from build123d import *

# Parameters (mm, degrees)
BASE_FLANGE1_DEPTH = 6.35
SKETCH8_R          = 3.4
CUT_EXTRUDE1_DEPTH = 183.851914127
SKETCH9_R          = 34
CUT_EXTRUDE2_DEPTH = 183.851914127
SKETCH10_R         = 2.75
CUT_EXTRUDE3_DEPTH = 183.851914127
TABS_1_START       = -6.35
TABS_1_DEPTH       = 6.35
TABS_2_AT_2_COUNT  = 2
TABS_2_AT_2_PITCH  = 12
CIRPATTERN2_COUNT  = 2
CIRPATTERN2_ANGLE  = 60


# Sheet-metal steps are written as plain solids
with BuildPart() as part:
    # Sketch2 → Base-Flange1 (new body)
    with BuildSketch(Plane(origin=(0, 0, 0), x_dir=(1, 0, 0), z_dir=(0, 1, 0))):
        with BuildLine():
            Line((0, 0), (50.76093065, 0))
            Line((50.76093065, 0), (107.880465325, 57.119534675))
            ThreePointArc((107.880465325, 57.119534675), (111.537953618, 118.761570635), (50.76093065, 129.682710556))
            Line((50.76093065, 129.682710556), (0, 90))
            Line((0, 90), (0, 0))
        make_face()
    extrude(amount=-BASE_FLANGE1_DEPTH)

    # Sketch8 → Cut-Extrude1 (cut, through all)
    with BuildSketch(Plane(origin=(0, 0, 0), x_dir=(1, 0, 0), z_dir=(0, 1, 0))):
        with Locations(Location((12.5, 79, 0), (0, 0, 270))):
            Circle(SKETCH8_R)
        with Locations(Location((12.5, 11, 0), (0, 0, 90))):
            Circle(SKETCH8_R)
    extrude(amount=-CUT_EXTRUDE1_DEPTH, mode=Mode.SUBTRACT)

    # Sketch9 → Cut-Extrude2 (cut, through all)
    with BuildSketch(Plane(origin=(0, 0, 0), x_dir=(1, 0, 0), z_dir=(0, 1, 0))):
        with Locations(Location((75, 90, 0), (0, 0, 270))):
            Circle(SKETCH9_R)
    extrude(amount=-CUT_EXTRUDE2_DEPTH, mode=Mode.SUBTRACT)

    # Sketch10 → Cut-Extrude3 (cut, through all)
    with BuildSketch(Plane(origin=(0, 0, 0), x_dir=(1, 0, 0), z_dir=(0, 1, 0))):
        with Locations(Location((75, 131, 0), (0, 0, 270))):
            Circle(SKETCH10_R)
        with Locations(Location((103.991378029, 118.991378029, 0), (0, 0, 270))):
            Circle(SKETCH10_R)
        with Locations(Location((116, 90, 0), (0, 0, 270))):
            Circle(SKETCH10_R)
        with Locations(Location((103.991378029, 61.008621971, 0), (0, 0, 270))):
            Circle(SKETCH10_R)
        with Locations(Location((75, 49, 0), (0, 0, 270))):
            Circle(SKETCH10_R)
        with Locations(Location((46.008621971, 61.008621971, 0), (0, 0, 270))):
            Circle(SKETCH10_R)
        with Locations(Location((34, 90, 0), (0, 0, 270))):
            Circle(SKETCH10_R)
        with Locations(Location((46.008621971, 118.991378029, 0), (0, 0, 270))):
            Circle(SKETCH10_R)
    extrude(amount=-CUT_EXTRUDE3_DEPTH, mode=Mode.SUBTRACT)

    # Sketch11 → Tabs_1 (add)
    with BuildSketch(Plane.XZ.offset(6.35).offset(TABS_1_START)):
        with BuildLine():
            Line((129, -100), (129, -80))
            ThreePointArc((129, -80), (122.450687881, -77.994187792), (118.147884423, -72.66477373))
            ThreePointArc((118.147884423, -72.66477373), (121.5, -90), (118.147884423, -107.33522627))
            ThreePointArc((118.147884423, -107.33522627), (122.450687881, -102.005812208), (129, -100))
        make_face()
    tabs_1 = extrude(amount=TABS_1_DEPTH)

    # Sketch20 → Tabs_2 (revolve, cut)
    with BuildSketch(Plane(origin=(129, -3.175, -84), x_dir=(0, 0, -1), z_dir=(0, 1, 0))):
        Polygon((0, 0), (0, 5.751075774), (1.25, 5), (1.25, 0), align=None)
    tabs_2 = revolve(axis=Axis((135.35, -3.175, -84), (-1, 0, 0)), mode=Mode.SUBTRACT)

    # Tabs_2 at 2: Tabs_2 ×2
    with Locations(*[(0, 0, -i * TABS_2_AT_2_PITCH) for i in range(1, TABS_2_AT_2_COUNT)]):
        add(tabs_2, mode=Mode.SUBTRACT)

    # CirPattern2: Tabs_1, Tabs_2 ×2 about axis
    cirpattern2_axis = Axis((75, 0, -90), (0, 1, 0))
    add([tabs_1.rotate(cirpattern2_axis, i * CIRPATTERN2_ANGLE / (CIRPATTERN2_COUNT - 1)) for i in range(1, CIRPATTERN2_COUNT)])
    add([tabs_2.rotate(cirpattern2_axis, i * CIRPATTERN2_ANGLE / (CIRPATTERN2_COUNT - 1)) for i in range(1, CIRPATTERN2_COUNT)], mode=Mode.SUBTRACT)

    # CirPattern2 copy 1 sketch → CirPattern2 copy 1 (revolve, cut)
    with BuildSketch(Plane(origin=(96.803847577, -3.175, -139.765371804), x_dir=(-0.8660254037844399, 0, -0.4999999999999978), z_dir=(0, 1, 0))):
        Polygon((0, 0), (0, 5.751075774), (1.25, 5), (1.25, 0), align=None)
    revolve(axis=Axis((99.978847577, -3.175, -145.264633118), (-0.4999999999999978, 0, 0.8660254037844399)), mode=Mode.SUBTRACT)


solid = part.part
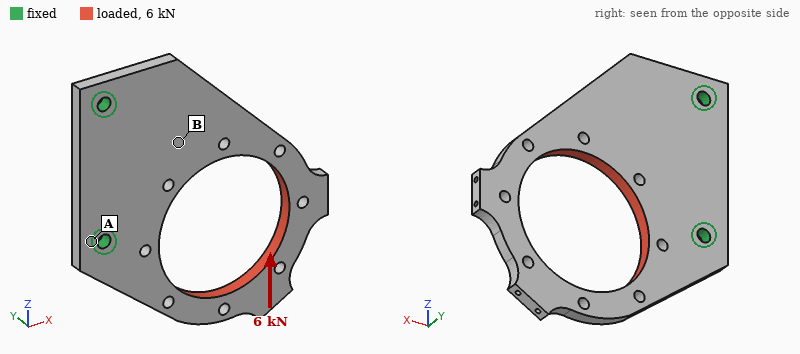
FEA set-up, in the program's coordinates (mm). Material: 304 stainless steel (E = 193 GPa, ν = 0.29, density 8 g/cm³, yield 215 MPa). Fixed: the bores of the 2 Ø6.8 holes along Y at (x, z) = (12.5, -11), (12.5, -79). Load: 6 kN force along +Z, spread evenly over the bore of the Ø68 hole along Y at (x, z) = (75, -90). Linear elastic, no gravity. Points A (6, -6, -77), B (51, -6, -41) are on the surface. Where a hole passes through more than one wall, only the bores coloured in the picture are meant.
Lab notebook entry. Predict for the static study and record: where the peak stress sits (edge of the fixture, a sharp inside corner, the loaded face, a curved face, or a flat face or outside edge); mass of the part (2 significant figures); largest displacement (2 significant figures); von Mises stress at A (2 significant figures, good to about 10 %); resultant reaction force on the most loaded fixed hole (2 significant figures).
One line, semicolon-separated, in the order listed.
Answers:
a curved face; 440 g; 0.11 mm; 28 MPa; 6.1 kN
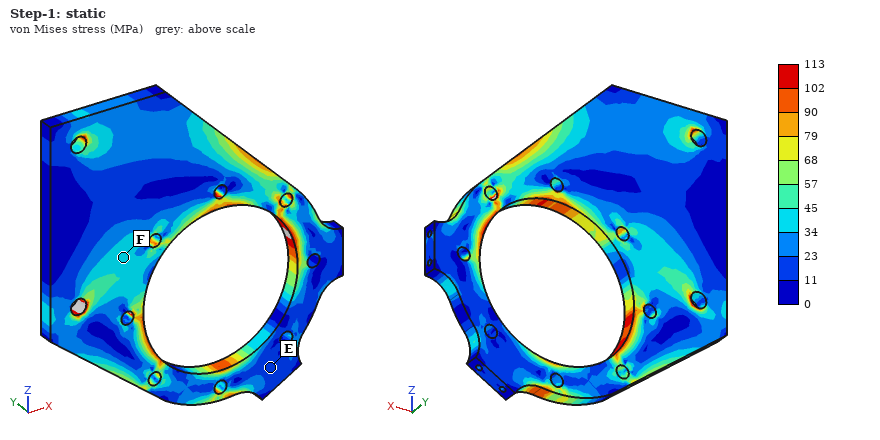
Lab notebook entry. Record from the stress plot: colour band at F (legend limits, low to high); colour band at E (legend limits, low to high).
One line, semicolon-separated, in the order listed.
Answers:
34 to 45 MPa; 11 to 23 MPa
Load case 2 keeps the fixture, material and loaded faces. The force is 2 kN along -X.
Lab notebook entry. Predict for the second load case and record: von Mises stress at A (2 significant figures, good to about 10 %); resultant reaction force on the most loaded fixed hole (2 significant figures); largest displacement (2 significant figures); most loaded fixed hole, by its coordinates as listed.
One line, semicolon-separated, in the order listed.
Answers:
12 MPa; 2.2 kN; 33 µm; (12.5, -79)
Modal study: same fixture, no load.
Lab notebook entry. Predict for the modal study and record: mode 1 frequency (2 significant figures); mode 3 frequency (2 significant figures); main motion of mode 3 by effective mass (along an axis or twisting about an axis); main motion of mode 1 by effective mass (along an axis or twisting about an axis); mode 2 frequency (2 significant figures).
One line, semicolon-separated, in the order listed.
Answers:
420 Hz; 1800 Hz; along Y; along Y; 950 Hz
